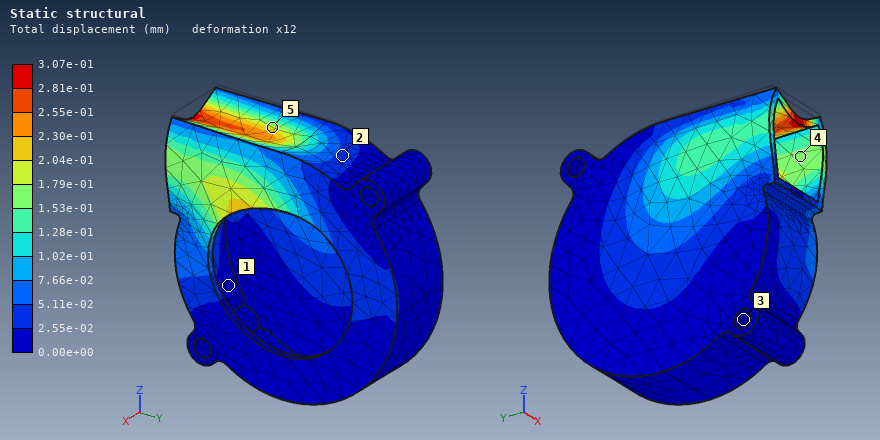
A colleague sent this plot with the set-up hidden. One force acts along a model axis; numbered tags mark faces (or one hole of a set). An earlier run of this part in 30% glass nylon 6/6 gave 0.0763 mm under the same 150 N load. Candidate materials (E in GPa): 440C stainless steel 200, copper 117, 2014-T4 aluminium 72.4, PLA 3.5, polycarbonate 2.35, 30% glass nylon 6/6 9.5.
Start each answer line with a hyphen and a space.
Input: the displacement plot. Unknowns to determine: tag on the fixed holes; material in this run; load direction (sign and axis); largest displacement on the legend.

- 3
- polycarbonate
- -Z
- 3.07e-01 mm
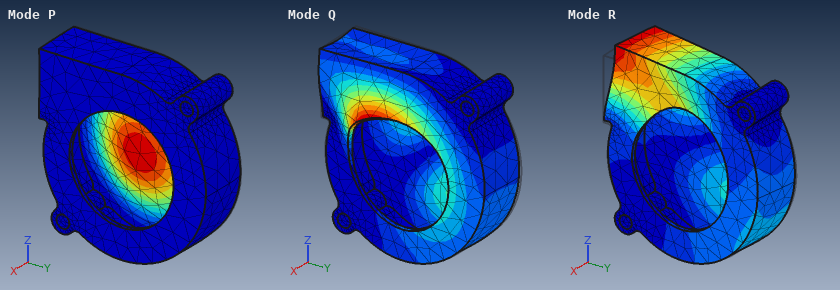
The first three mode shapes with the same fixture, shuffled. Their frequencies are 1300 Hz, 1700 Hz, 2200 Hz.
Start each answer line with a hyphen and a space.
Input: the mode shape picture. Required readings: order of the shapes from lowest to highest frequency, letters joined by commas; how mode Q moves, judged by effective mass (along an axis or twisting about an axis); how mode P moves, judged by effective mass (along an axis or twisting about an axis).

- P, R, Q
- along X
- along X
